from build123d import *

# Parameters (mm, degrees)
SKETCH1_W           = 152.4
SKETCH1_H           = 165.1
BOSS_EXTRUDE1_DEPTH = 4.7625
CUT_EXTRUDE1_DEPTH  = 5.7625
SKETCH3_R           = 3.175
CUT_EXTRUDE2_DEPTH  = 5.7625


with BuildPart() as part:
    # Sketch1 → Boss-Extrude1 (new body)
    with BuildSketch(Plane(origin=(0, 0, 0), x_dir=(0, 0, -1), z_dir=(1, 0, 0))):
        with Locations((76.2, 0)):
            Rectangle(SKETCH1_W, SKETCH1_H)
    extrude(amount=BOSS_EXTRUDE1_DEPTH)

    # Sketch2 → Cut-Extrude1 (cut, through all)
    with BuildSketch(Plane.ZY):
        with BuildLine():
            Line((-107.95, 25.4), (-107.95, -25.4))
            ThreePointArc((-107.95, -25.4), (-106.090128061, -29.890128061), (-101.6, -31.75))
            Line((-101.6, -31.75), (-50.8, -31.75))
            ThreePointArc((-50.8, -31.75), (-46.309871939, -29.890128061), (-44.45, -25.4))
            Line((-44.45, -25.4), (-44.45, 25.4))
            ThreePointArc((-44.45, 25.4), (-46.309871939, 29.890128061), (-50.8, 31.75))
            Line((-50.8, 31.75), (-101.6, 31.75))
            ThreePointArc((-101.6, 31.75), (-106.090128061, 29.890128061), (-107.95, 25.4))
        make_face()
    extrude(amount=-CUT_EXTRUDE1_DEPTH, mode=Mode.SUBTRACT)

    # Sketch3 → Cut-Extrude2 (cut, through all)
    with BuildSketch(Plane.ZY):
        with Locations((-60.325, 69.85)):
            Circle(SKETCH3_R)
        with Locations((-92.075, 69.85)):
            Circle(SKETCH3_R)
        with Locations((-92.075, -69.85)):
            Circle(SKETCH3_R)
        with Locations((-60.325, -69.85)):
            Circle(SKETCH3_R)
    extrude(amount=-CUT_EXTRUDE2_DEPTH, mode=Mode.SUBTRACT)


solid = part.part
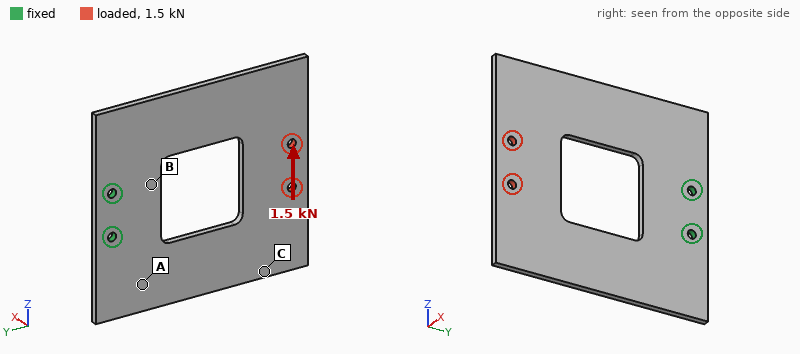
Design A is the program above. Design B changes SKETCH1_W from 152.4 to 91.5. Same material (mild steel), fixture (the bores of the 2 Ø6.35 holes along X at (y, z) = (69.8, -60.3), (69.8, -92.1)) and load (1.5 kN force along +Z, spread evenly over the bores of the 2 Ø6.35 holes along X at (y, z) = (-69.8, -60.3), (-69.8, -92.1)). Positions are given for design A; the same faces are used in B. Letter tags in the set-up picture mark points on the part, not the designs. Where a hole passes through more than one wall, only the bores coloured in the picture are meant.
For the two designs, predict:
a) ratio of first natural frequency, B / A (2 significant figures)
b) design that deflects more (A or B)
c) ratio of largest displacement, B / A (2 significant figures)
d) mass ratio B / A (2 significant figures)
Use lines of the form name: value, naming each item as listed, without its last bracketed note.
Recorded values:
ratio of first natural frequency, B / A: 0.96
design that deflects more: B
ratio of largest displacement, B / A: 2.1
mass ratio B / A: 0.52
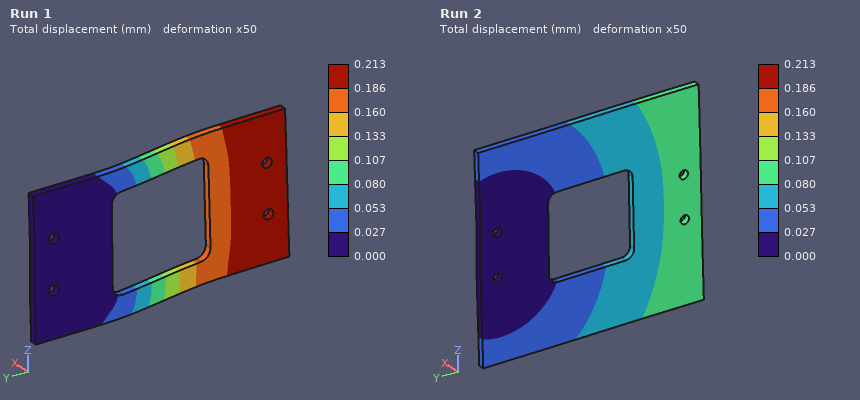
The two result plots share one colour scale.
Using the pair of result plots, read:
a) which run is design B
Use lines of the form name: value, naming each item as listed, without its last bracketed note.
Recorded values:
which run is design B: Run 1
